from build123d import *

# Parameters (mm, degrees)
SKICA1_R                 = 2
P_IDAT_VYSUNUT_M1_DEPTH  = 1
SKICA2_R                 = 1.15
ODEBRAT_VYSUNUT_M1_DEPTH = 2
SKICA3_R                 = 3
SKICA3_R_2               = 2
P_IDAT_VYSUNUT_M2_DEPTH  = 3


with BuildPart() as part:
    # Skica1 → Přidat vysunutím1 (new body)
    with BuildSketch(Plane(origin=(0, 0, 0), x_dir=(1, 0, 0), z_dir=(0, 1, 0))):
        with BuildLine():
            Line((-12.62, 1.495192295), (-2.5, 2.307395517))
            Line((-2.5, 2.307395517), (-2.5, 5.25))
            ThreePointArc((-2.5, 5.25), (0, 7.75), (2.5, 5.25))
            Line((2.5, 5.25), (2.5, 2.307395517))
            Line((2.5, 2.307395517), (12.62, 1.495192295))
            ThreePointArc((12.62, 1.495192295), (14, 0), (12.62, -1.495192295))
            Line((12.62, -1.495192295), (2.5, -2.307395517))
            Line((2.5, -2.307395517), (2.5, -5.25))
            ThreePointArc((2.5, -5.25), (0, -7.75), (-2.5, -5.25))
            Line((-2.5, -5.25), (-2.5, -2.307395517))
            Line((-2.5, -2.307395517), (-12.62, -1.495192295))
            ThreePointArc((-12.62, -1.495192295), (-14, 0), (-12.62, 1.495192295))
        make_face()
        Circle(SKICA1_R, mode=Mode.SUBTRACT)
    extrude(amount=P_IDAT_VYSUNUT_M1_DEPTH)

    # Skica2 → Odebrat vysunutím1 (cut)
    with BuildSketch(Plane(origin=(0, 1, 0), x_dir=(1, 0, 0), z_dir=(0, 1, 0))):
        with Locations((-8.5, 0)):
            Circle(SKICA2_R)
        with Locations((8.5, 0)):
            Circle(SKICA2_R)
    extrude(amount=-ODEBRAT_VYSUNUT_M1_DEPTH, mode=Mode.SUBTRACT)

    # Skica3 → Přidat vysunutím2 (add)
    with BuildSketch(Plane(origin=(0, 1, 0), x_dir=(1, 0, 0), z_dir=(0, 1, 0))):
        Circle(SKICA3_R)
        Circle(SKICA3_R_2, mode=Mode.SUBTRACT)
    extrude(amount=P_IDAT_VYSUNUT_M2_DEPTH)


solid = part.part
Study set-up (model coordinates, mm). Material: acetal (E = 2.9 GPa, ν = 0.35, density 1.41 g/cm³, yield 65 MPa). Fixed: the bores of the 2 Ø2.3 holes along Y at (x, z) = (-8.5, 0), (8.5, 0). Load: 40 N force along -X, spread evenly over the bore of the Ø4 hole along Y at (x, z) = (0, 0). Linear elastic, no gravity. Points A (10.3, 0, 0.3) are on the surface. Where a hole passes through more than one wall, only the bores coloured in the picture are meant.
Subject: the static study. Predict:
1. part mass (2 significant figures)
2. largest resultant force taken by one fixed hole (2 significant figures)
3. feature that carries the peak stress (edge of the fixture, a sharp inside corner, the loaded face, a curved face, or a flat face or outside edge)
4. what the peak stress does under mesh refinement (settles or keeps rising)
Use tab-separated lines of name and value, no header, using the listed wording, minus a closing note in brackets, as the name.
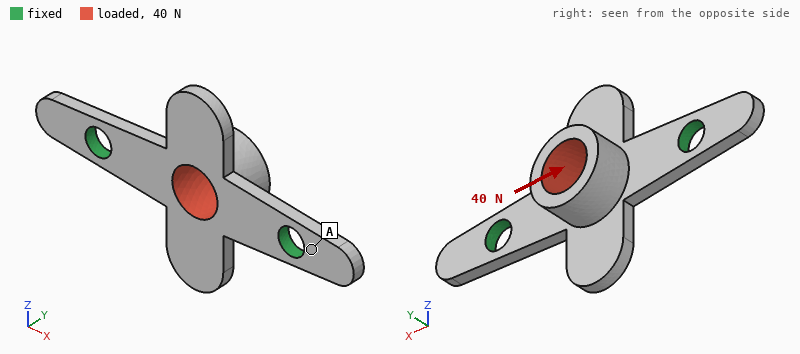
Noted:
part mass	0.26 g
largest resultant force taken by one fixed hole	21 N
feature that carries the peak stress	edge of the fixture
what the peak stress does under mesh refinement	keeps rising
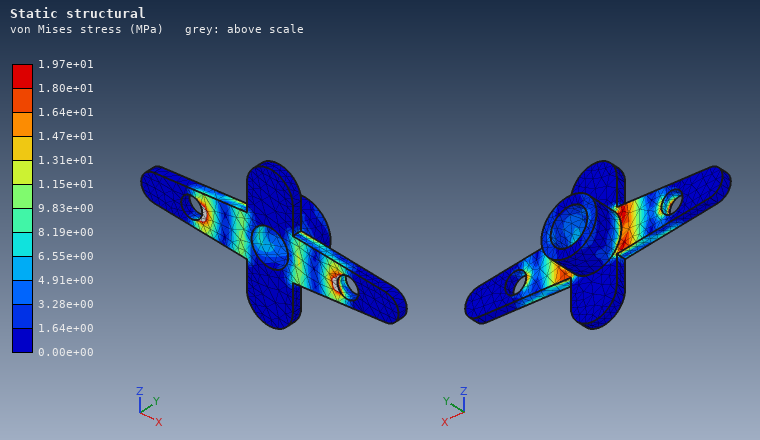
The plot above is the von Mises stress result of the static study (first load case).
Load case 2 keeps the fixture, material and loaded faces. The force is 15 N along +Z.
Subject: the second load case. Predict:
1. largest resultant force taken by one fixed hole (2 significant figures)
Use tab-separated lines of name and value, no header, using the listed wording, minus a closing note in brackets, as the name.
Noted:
largest resultant force taken by one fixed hole	7.5 N
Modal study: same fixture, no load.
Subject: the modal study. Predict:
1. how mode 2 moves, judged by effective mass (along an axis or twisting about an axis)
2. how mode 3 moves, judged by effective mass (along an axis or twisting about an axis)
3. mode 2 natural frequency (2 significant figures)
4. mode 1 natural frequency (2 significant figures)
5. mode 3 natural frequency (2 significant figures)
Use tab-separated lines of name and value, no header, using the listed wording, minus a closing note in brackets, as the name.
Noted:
how mode 2 moves, judged by effective mass	along Y
how mode 3 moves, judged by effective mass	along Z
mode 2 natural frequency	4000 Hz
mode 1 natural frequency	2500 Hz
mode 3 natural frequency	9900 Hz
